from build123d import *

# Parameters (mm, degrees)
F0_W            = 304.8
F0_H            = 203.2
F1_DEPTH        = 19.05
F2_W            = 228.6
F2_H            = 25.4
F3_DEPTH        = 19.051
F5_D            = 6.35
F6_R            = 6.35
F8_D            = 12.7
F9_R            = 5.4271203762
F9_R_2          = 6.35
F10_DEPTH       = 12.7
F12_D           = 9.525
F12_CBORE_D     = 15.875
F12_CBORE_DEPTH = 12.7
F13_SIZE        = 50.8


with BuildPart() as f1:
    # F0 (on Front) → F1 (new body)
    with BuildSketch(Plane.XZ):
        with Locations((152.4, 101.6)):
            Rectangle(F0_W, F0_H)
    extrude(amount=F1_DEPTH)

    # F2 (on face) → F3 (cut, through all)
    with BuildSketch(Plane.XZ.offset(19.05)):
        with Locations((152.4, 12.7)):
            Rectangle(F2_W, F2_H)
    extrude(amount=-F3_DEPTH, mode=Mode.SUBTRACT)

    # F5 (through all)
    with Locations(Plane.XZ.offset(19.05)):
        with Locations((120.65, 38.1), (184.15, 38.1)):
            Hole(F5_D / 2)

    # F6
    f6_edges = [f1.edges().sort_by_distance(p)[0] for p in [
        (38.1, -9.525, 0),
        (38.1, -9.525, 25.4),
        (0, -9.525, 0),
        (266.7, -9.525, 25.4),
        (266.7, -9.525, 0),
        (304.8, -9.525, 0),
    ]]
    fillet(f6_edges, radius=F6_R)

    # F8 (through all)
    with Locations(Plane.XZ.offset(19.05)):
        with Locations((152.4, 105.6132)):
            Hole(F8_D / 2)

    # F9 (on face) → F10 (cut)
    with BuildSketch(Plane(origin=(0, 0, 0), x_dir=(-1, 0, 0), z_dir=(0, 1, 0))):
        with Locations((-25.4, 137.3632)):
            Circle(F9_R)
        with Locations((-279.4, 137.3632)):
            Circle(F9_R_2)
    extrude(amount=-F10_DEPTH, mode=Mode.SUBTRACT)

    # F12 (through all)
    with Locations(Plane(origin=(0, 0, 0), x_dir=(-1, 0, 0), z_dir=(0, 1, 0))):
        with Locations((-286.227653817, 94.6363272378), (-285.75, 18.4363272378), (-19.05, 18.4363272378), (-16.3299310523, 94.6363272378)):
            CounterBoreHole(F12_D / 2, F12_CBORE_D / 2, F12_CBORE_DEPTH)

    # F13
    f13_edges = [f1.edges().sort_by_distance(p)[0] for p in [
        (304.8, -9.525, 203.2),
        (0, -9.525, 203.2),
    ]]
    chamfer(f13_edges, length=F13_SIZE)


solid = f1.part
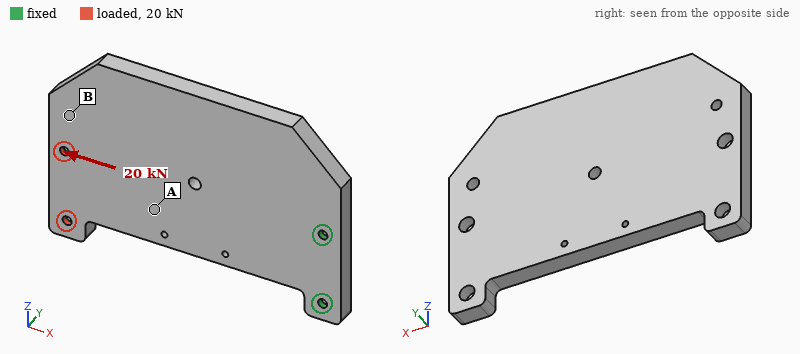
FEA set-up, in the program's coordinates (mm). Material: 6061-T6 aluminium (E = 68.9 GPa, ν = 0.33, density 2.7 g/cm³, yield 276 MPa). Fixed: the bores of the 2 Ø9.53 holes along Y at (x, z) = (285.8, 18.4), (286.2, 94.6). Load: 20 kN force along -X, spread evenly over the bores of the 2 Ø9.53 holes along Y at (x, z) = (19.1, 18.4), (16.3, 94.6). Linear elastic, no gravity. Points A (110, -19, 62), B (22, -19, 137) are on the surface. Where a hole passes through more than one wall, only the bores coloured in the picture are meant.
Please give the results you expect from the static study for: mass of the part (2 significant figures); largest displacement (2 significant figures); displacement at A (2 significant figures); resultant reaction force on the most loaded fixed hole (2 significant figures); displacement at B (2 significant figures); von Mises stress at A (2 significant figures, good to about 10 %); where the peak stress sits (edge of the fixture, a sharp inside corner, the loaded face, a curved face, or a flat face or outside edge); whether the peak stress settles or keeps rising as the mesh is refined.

2.7 kg
0.89 mm
0.34 mm
10 kN
0.73 mm
27 MPa
edge of the fixture
keeps rising
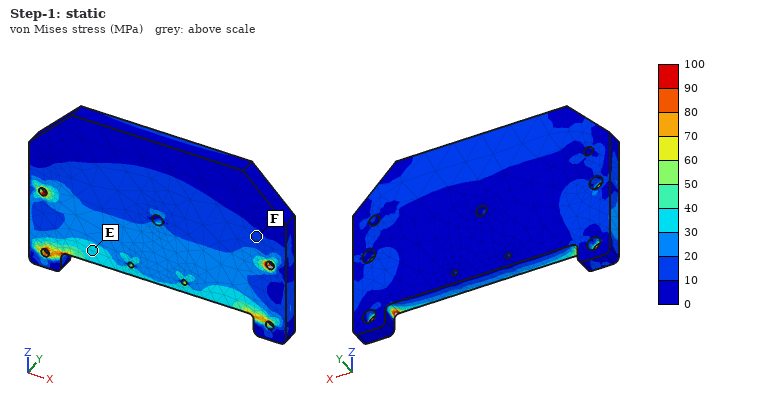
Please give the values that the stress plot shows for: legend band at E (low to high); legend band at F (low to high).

30 to 40 MPa
10 to 20 MPa
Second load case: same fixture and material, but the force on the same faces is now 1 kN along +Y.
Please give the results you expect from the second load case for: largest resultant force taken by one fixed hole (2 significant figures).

1.5 kN
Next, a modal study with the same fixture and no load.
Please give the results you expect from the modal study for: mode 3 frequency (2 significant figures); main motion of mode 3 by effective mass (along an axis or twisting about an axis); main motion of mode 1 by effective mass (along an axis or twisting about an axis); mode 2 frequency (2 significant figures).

590 Hz
along Z
along Y
450 Hz
